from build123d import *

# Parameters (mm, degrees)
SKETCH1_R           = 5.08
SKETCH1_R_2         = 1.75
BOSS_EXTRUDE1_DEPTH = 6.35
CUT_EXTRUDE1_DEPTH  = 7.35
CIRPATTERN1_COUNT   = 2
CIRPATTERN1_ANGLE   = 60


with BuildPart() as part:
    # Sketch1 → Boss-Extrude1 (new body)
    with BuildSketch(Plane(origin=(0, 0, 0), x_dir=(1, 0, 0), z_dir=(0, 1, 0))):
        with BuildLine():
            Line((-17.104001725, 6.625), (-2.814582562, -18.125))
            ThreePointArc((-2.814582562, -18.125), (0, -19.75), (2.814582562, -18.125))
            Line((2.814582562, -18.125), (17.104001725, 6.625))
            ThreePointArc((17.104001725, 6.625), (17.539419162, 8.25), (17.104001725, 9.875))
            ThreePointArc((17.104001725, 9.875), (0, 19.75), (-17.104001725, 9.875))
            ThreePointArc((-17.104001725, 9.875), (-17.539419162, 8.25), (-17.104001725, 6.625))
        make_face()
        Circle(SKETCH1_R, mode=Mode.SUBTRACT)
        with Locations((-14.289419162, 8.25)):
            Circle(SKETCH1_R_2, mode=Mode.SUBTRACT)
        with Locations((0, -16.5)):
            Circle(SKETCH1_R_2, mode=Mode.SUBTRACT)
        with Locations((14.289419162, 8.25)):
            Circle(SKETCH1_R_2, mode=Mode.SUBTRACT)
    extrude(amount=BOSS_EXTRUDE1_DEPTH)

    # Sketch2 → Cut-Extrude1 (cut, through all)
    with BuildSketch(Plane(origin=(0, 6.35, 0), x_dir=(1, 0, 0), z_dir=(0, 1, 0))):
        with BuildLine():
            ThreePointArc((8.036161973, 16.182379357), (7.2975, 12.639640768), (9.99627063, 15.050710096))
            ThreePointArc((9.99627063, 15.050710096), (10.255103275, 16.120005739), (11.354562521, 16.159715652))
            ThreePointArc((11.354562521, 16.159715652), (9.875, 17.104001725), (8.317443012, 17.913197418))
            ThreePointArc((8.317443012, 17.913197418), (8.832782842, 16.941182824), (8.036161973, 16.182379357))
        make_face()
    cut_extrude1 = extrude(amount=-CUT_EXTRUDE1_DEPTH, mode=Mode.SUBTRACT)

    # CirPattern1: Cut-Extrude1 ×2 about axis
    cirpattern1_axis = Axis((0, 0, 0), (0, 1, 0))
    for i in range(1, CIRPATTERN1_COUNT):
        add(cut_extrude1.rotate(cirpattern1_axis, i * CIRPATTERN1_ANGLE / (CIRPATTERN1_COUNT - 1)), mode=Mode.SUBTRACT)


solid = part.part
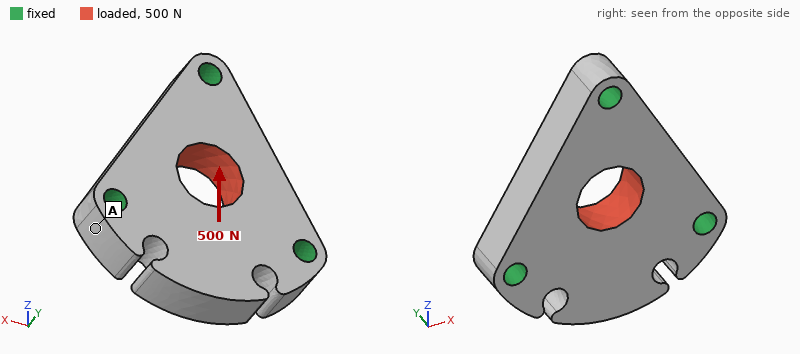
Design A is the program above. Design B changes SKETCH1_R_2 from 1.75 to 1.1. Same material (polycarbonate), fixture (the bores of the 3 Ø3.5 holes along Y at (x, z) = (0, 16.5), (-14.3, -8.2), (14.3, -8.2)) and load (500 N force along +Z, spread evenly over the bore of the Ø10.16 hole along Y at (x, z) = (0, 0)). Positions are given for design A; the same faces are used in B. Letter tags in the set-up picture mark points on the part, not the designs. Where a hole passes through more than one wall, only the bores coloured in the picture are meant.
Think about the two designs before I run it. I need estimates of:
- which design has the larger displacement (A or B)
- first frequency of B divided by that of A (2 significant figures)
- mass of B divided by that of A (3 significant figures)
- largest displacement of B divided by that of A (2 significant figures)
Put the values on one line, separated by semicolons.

B; 0.93; 1.02; 1.2
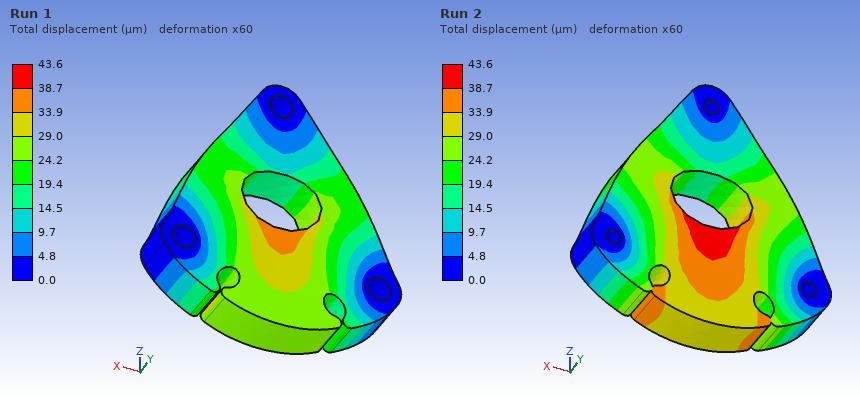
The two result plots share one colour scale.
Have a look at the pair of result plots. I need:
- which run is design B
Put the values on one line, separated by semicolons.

Run 2
